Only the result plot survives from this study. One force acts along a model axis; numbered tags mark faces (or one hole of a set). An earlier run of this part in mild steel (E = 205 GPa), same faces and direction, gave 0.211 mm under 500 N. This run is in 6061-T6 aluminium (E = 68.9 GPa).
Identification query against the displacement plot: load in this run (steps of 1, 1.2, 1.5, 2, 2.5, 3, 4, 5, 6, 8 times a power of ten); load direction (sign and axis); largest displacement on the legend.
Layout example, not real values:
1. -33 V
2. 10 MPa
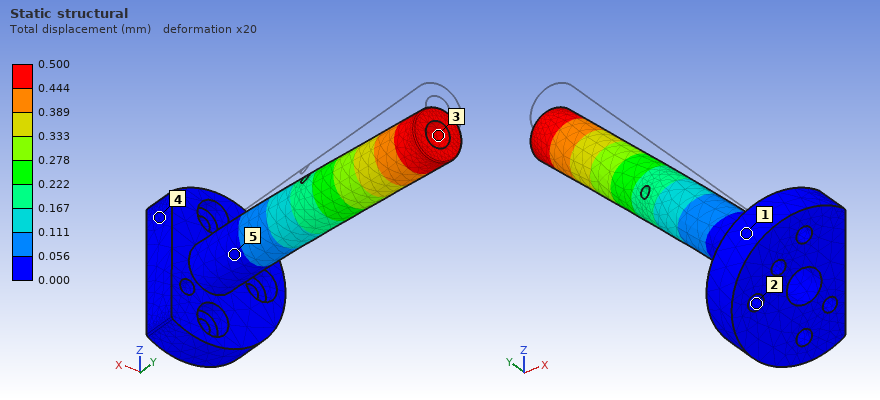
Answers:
1. 400 N
2. -Z
3. 0.500 mm
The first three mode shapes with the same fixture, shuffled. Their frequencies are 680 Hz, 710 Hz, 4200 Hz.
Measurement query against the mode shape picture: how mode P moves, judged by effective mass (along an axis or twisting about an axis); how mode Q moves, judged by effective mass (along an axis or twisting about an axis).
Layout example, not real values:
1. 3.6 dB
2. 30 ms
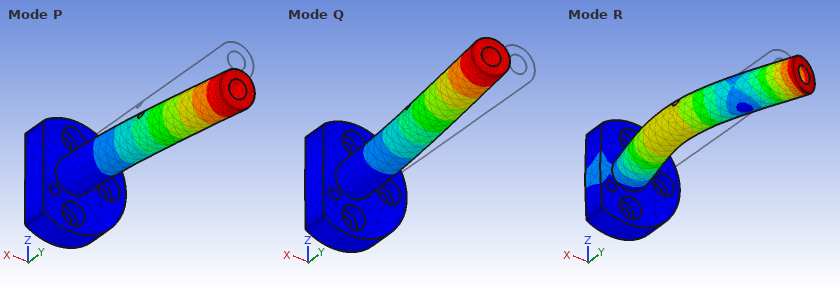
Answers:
1. along Z
2. along X
